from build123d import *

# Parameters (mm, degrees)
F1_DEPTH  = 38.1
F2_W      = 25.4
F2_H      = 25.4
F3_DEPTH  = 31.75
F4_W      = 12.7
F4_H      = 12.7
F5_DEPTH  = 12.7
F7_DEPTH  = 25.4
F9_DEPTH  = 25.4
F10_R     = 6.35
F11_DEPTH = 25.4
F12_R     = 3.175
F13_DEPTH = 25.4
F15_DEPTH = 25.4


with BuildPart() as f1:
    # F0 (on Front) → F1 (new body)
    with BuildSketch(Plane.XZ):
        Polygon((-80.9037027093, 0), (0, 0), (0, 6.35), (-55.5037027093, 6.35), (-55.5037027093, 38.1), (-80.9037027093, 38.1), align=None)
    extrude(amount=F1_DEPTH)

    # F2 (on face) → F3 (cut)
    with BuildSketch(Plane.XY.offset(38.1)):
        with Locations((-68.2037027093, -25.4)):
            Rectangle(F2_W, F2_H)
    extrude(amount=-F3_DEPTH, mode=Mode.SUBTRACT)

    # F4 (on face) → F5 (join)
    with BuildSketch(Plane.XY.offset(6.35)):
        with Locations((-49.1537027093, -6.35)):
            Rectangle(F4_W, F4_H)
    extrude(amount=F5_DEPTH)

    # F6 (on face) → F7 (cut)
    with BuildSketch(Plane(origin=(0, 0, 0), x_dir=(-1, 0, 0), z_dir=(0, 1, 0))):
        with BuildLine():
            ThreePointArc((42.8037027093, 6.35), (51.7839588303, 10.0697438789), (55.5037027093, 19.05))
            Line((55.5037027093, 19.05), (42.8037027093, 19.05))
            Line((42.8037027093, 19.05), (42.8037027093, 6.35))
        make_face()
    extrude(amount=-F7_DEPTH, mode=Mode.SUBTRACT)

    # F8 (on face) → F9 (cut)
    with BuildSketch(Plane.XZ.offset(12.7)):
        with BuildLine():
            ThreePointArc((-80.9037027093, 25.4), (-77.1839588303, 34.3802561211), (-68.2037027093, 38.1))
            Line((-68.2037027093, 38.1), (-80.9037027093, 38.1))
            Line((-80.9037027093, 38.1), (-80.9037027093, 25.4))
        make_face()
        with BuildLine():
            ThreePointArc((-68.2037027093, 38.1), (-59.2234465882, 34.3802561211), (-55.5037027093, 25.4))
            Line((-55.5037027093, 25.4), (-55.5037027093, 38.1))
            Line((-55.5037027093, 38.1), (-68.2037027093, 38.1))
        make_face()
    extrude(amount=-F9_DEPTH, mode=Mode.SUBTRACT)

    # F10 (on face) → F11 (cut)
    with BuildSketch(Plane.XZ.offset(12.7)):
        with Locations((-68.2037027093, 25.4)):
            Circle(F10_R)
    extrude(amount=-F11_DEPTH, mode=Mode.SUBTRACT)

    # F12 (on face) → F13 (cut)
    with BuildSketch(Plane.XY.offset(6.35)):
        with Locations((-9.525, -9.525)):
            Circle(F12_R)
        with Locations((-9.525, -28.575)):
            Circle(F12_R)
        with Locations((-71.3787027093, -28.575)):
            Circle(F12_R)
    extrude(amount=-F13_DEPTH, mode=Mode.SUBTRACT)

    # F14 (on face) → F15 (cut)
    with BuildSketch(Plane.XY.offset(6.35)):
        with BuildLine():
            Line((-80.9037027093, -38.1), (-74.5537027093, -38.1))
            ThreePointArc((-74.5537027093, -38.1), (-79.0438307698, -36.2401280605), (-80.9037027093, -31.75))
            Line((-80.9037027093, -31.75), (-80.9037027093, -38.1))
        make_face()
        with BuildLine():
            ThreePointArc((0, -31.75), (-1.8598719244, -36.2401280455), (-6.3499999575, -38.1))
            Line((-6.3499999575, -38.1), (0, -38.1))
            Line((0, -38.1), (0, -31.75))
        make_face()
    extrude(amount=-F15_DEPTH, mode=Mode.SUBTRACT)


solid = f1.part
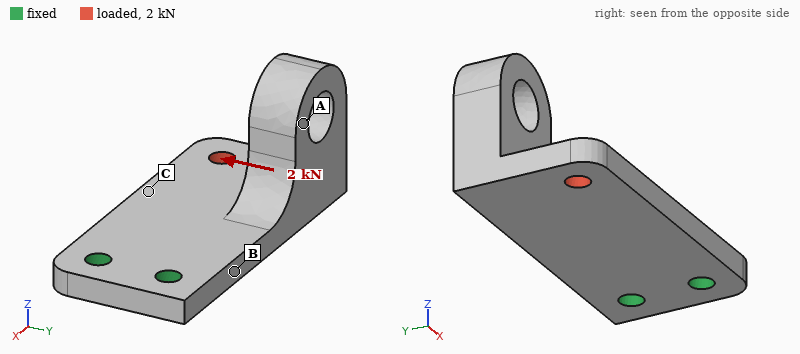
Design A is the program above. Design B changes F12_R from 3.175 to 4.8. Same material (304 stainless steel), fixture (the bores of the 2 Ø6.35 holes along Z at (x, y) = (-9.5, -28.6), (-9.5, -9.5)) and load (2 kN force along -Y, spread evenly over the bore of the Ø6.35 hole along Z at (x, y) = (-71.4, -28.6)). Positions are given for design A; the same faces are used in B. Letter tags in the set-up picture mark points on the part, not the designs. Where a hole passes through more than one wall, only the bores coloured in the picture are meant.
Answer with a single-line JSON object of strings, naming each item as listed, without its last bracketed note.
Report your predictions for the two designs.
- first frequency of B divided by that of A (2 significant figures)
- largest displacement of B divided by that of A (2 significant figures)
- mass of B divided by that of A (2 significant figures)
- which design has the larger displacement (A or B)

{"first frequency of B divided by that of A": "1.1", "largest displacement of B divided by that of A": "0.88", "mass of B divided by that of A": "0.97", "which design has the larger displacement": "A"}
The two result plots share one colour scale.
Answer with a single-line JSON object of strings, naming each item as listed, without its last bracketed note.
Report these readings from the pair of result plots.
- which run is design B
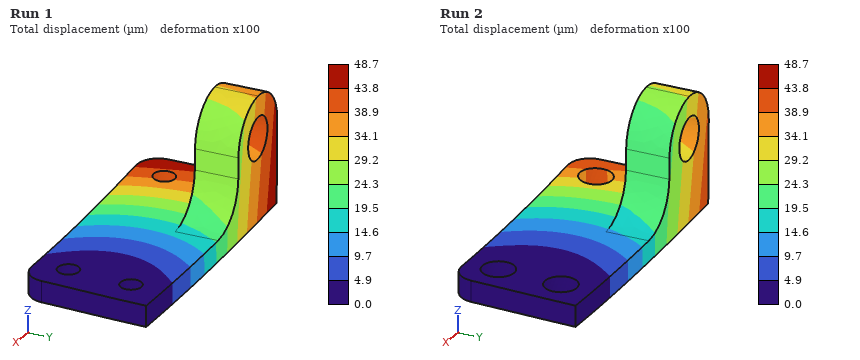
{"which run is design B": "Run 2"}
